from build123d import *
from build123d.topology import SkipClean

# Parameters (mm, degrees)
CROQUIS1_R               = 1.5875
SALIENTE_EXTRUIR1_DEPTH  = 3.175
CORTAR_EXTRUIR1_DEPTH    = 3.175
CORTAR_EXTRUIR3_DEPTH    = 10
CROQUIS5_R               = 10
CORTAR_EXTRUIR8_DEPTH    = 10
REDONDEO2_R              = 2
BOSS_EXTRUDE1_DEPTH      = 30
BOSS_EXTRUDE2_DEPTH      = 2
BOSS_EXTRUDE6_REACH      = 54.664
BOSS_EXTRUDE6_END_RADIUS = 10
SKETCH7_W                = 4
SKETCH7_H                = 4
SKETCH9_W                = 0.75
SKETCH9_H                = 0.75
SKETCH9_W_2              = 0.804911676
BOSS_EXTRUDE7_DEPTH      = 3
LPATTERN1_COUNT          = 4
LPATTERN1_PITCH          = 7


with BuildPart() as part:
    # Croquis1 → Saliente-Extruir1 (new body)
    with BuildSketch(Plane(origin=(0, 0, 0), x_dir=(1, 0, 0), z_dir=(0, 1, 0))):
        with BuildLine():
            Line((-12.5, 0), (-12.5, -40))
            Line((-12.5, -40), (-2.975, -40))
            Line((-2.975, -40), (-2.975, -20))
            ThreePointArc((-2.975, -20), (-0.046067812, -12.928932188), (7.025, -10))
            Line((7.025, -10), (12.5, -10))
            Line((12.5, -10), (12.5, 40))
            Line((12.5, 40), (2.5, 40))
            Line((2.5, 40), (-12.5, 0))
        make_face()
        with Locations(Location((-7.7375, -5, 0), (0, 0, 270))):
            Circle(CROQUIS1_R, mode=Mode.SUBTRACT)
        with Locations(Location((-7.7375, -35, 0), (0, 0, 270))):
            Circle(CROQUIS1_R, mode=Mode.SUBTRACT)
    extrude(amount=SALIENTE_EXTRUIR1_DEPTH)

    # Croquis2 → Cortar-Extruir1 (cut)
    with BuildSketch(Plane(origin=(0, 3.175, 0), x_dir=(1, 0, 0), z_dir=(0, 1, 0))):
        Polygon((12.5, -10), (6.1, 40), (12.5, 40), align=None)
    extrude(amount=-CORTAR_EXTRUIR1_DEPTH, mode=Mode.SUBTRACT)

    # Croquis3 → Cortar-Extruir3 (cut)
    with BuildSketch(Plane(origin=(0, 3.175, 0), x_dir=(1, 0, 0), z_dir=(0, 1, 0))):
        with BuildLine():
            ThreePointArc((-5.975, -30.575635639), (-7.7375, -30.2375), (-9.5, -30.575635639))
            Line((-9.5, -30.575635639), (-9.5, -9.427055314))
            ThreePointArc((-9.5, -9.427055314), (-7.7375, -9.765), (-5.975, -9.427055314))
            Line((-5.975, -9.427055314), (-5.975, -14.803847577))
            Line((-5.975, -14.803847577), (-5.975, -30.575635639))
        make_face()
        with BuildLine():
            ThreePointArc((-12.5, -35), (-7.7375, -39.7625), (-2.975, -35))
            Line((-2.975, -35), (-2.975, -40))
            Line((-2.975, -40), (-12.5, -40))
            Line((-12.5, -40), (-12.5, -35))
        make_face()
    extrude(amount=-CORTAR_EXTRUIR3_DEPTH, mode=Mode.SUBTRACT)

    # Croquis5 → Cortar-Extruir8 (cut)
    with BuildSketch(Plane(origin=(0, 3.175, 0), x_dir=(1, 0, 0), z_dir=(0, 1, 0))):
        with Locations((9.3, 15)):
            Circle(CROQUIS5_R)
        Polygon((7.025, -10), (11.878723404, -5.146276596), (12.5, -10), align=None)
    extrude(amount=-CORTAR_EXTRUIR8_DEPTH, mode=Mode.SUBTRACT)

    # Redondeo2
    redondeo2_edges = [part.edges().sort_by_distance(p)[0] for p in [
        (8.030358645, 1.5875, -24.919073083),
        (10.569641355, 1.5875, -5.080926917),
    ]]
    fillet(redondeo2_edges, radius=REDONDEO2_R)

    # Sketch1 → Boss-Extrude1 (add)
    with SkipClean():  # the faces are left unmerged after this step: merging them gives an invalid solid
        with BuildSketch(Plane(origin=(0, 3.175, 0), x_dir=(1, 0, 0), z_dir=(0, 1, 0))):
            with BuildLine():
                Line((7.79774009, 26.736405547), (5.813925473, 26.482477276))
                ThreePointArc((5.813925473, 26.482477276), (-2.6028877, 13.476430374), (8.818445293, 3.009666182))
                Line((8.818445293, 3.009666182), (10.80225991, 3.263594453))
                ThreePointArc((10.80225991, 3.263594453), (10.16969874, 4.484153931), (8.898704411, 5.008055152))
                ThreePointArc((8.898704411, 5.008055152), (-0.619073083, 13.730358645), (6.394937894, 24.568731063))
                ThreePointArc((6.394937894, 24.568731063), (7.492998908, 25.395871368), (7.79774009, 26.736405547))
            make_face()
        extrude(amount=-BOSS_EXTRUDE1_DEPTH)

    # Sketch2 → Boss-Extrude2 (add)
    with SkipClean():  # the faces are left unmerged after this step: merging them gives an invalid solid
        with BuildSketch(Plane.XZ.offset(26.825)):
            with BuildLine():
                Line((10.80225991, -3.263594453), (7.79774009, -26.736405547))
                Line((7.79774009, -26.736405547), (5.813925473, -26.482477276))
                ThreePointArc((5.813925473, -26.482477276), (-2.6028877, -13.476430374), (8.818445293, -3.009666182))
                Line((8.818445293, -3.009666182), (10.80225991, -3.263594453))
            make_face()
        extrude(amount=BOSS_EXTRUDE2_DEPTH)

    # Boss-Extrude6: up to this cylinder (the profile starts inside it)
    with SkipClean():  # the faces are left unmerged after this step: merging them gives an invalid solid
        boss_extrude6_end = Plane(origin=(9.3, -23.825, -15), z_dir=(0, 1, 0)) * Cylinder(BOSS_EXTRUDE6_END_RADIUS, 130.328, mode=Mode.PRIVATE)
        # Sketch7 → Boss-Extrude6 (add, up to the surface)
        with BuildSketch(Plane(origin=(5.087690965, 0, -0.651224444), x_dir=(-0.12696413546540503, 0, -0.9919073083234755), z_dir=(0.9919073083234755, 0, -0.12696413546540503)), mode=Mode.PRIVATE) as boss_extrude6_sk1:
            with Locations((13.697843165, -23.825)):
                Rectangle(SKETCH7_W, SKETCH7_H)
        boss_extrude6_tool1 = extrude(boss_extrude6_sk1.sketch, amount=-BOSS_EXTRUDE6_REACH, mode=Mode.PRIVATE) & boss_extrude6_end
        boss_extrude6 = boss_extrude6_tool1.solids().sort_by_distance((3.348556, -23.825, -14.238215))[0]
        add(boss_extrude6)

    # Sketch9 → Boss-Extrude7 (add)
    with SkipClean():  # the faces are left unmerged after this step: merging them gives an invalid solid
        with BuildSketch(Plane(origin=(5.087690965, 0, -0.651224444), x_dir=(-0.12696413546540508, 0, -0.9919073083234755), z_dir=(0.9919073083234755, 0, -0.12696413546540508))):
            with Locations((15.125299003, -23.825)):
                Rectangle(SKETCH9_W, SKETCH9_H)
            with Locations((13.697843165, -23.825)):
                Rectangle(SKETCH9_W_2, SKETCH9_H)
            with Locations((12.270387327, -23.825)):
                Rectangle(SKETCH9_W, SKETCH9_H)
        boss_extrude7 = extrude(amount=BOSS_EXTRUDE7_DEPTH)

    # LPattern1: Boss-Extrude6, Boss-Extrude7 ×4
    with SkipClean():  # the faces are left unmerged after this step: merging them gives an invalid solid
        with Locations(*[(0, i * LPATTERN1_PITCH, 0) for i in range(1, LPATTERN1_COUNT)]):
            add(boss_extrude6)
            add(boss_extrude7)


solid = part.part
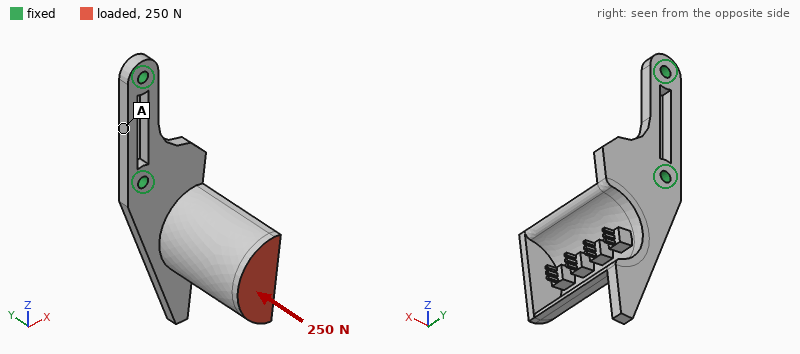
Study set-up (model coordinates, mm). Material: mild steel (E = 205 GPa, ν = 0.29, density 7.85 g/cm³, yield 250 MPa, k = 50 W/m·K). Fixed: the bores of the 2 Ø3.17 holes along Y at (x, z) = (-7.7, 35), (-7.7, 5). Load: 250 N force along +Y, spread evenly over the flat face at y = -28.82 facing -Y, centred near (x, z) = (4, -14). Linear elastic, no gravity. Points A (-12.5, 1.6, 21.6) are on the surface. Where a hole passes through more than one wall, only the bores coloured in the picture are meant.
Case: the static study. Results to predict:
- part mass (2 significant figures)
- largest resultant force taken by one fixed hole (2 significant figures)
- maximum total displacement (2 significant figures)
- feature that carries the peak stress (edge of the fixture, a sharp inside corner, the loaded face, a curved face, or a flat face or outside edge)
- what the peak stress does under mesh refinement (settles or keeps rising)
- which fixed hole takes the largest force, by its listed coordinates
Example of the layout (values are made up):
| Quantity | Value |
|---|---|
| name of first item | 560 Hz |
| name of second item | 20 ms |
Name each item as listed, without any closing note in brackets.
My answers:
| Quantity | Value |
|---|---|
| part mass | 40 g |
| largest resultant force taken by one fixed hole | 280 N |
| maximum total displacement | 0.28 mm |
| feature that carries the peak stress | edge of the fixture |
| what the peak stress does under mesh refinement | keeps rising |
| which fixed hole takes the largest force, by its listed coordinates | (-7.7, 5) |
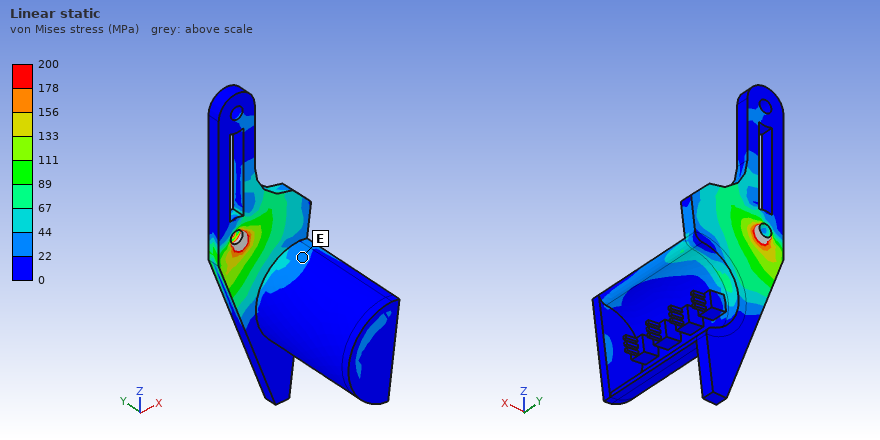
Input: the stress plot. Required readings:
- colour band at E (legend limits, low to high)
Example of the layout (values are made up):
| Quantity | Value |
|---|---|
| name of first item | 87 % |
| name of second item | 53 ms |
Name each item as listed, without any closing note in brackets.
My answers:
| Quantity | Value |
|---|---|
| colour band at E | 22 to 44 MPa |
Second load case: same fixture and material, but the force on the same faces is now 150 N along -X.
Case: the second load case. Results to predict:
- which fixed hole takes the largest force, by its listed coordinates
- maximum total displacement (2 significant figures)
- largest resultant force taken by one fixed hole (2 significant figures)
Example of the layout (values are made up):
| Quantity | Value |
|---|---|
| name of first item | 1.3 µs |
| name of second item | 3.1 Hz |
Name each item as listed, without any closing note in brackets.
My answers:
| Quantity | Value |
|---|---|
| which fixed hole takes the largest force, by its listed coordinates | (-7.7, 5) |
| maximum total displacement | 0.27 mm |
| largest resultant force taken by one fixed hole | 180 N |
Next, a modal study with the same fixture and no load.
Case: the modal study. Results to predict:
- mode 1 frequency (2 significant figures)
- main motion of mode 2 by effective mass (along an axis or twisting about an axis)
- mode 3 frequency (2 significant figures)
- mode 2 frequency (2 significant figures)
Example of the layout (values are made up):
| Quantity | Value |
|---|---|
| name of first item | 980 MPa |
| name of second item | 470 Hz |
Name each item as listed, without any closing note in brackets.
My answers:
| Quantity | Value |
|---|---|
| mode 1 frequency | 930 Hz |
| main motion of mode 2 by effective mass | along X |
| mode 3 frequency | 3400 Hz |
| mode 2 frequency | 1500 Hz |
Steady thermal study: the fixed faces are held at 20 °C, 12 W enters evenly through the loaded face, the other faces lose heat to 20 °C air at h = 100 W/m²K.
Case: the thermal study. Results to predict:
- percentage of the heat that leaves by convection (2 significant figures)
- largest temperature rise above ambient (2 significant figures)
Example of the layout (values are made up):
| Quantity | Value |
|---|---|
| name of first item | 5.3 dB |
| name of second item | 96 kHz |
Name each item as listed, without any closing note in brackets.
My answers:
| Quantity | Value |
|---|---|
| percentage of the heat that leaves by convection | 86 % |
| largest temperature rise above ambient | 73 K |
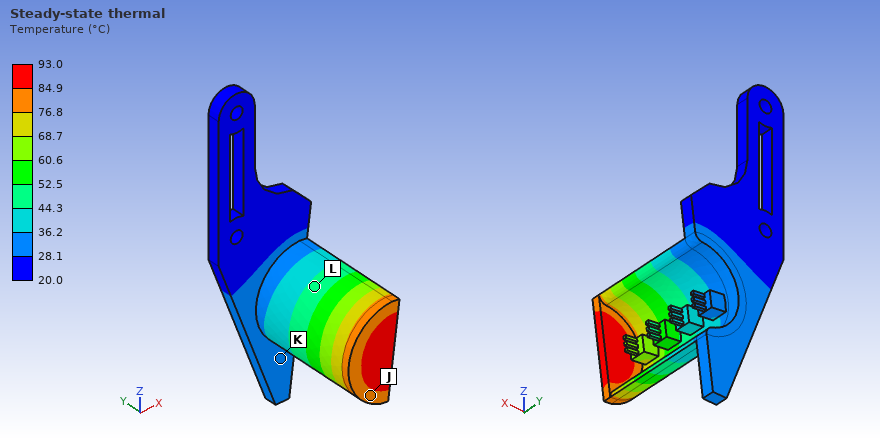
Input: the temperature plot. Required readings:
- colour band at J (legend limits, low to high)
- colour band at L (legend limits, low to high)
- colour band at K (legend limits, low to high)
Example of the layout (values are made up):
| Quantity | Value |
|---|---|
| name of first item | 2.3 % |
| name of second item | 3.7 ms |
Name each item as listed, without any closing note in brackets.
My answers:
| Quantity | Value |
|---|---|
| colour band at J | 76.8 to 84.9 °C |
| colour band at L | 44.3 to 52.5 °C |
| colour band at K | 28.1 to 36.2 °C |
